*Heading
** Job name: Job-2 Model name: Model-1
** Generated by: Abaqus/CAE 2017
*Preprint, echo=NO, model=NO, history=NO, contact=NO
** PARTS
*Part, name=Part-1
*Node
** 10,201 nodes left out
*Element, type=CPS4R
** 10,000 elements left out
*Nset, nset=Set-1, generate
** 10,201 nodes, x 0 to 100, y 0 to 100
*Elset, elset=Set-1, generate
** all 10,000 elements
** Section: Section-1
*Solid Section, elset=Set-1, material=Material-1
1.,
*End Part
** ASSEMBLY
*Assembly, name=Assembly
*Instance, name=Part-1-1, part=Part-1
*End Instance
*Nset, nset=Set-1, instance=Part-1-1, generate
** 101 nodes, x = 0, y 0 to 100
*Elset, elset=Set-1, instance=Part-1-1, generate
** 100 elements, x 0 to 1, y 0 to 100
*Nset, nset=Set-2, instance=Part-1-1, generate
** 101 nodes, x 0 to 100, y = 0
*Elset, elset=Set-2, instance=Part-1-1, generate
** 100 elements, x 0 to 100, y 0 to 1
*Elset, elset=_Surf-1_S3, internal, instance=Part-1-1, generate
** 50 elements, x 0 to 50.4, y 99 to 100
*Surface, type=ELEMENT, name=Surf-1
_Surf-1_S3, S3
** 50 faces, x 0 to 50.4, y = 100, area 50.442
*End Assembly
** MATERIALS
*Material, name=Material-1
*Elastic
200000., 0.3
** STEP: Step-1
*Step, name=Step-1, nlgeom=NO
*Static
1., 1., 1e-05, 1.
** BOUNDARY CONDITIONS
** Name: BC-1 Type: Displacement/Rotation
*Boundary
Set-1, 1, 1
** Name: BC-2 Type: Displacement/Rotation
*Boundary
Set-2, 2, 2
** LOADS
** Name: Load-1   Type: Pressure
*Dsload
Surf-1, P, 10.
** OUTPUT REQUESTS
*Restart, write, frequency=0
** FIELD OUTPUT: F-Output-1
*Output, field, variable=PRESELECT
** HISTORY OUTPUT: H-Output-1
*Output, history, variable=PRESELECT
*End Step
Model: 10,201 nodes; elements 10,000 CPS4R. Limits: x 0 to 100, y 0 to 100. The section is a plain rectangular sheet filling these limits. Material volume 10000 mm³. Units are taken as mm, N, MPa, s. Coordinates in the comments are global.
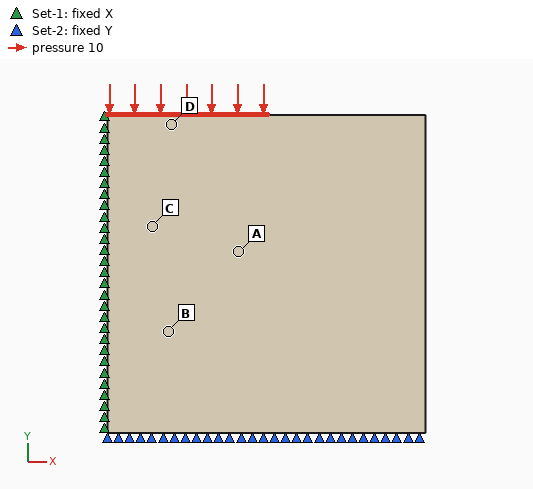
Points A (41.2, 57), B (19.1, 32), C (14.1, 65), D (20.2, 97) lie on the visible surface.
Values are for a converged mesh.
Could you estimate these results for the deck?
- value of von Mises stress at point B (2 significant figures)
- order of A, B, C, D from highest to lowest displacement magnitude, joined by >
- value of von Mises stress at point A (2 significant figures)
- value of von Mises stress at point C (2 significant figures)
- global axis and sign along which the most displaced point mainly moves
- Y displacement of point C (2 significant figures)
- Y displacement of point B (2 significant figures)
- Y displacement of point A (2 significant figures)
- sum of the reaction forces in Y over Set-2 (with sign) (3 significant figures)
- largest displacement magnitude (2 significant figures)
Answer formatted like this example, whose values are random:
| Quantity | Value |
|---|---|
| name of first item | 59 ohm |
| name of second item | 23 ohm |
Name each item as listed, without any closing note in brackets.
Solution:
| Quantity | Value |
|---|---|
| value of von Mises stress at point B | 8.9 MPa |
| order of A, B, C, D from highest to lowest displacement magnitude, joined by > | D > C > A > B |
| value of von Mises stress at point A | 7.3 MPa |
| value of von Mises stress at point C | 9.3 MPa |
| global axis and sign along which the most displaced point mainly moves | -Y |
| Y displacement of point C | -0.0028 mm |
| Y displacement of point B | -0.0013 mm |
| Y displacement of point A | -0.0019 mm |
| sum of the reaction forces in Y over Set-2 (with sign) | 504 N |
| largest displacement magnitude | 0.0045 mm |
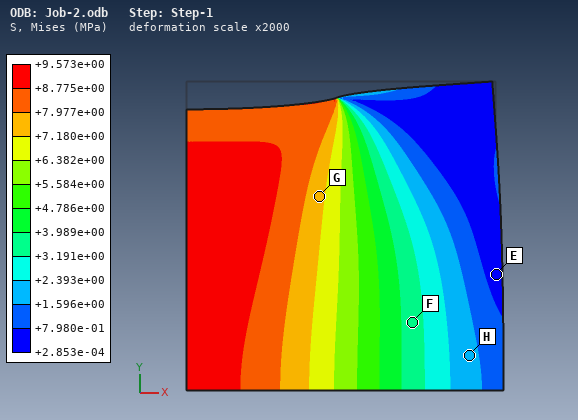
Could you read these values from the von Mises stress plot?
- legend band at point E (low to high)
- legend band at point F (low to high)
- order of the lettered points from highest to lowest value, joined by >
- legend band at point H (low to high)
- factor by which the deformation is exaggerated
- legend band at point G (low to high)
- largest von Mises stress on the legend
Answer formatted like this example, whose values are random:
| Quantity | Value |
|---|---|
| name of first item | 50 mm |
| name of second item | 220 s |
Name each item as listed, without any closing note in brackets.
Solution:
| Quantity | Value |
|---|---|
| legend band at point E | +2.853e-04 to +7.980e-01 MPa |
| legend band at point F | +3.191e+00 to +3.989e+00 MPa |
| order of the lettered points from highest to lowest value, joined by > | G > F > H > E |
| legend band at point H | +1.596e+00 to +2.393e+00 MPa |
| factor by which the deformation is exaggerated | 2000 |
| legend band at point G | +7.180e+00 to +7.977e+00 MPa |
| largest von Mises stress on the legend | +9.573e+00 MPa |
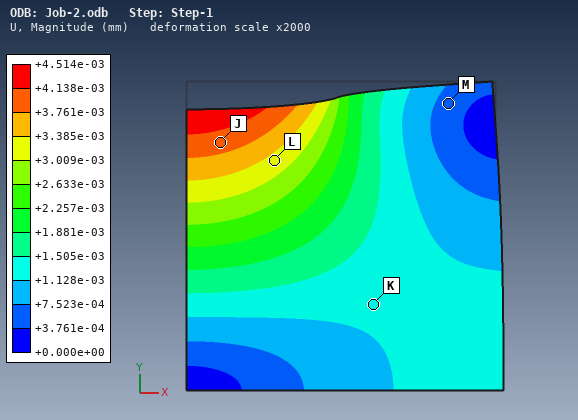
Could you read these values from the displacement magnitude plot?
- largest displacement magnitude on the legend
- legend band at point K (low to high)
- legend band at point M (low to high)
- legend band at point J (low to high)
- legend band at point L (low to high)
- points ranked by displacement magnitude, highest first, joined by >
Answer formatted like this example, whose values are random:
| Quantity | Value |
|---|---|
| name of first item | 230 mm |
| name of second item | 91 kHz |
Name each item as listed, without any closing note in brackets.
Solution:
| Quantity | Value |
|---|---|
| largest displacement magnitude on the legend | +4.514e-03 mm |
| legend band at point K | +1.128e-03 to +1.505e-03 mm |
| legend band at point M | +3.761e-04 to +7.523e-04 mm |
| legend band at point J | +3.761e-03 to +4.138e-03 mm |
| legend band at point L | +3.009e-03 to +3.385e-03 mm |
| points ranked by displacement magnitude, highest first, joined by > | J > L > K > M |
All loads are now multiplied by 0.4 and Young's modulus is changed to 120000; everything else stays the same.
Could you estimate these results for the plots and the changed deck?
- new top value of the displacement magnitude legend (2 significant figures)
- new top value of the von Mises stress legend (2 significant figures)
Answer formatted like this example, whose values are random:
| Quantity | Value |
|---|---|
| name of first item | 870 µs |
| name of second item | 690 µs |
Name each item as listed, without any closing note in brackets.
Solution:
| Quantity | Value |
|---|---|
| new top value of the displacement magnitude legend | 0.0030 mm |
| new top value of the von Mises stress legend | 3.8 MPa |
